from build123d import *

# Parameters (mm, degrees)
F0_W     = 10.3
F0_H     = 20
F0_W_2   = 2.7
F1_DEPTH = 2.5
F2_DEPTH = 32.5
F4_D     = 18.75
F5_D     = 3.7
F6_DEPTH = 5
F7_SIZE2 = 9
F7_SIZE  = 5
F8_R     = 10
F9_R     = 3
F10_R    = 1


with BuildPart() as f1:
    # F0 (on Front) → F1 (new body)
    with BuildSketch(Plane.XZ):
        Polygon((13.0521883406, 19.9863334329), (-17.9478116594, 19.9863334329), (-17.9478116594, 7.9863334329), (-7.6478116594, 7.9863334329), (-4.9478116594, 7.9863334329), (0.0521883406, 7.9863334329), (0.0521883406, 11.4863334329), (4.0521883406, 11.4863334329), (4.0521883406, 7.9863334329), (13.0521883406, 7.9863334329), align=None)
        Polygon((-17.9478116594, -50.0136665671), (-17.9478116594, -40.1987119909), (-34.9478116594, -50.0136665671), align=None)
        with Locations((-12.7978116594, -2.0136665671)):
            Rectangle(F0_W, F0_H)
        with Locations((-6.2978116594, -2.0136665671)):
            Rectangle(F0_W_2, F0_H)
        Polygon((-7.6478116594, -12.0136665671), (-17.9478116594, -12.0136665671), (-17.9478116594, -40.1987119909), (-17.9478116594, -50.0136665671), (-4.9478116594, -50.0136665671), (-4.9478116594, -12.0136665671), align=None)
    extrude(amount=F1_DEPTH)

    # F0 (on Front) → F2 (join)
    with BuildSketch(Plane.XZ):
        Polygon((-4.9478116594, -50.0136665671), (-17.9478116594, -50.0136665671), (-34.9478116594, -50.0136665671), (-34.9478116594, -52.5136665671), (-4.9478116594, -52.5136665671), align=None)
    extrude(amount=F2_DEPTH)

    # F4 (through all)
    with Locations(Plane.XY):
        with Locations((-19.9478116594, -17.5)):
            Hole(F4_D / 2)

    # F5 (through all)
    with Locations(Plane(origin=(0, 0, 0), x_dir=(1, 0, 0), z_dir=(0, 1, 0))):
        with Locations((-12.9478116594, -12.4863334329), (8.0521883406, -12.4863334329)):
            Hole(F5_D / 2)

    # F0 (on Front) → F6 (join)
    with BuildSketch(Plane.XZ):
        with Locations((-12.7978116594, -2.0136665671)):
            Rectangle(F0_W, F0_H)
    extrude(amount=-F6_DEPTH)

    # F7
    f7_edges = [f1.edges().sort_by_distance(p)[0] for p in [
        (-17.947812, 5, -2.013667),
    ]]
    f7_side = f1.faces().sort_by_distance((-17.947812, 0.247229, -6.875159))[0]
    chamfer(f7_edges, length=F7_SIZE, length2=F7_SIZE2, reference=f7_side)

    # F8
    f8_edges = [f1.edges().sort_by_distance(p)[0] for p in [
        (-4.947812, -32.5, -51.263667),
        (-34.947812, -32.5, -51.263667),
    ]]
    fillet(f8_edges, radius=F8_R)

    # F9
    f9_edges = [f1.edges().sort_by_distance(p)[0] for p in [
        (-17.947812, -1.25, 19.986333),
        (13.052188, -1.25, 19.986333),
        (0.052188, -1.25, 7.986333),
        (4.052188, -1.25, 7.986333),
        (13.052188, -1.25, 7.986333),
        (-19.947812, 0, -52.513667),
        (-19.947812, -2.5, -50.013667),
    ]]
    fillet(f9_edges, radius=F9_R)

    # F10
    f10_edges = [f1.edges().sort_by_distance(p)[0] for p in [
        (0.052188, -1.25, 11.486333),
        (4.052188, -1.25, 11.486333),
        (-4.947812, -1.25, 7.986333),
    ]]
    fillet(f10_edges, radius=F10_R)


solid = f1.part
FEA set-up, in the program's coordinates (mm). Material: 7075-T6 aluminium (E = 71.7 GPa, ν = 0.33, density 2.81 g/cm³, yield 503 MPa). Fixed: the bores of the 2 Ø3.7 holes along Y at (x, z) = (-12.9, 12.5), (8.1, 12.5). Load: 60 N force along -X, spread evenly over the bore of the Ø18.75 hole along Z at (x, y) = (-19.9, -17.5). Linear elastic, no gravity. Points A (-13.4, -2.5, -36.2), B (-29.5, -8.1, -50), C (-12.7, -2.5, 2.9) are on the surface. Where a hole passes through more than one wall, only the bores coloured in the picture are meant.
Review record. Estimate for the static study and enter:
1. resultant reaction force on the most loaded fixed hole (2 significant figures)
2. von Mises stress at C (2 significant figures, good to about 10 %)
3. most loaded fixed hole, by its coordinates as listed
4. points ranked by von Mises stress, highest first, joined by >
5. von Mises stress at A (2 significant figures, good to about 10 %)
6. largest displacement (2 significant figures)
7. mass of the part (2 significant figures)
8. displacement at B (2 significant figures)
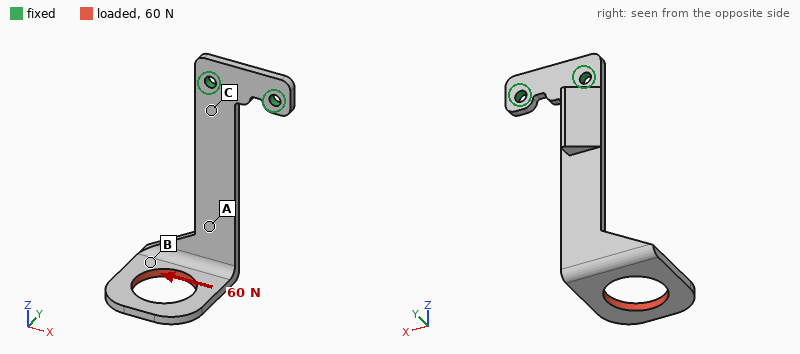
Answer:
160 N
31 MPa
(-12.9, 12.5)
A > C > B
74 MPa
0.99 mm
14 g
0.53 mm
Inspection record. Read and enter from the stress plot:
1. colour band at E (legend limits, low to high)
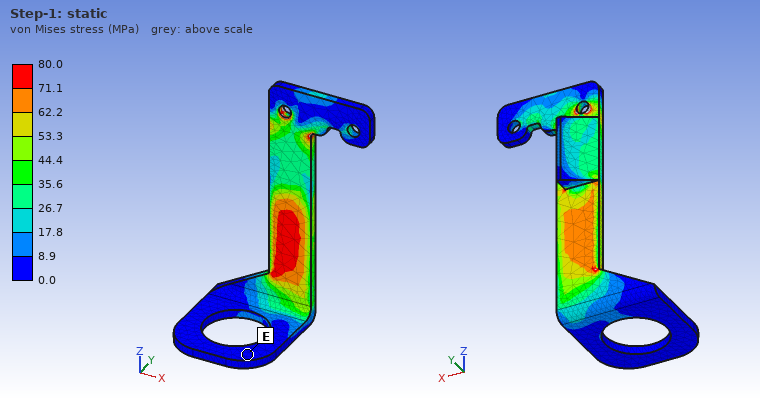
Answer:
0.0 to 8.9 MPa
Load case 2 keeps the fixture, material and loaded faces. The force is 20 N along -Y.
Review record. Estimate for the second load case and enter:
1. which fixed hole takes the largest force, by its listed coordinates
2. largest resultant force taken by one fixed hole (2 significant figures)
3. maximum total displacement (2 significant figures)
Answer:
(-12.9, 12.5)
31 N
1.0 mm
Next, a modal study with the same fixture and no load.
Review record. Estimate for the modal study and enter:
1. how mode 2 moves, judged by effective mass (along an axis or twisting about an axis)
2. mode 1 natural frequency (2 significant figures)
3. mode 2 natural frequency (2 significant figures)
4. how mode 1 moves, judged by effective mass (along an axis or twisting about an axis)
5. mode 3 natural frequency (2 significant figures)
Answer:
along X
310 Hz
690 Hz
along Y
1100 Hz
